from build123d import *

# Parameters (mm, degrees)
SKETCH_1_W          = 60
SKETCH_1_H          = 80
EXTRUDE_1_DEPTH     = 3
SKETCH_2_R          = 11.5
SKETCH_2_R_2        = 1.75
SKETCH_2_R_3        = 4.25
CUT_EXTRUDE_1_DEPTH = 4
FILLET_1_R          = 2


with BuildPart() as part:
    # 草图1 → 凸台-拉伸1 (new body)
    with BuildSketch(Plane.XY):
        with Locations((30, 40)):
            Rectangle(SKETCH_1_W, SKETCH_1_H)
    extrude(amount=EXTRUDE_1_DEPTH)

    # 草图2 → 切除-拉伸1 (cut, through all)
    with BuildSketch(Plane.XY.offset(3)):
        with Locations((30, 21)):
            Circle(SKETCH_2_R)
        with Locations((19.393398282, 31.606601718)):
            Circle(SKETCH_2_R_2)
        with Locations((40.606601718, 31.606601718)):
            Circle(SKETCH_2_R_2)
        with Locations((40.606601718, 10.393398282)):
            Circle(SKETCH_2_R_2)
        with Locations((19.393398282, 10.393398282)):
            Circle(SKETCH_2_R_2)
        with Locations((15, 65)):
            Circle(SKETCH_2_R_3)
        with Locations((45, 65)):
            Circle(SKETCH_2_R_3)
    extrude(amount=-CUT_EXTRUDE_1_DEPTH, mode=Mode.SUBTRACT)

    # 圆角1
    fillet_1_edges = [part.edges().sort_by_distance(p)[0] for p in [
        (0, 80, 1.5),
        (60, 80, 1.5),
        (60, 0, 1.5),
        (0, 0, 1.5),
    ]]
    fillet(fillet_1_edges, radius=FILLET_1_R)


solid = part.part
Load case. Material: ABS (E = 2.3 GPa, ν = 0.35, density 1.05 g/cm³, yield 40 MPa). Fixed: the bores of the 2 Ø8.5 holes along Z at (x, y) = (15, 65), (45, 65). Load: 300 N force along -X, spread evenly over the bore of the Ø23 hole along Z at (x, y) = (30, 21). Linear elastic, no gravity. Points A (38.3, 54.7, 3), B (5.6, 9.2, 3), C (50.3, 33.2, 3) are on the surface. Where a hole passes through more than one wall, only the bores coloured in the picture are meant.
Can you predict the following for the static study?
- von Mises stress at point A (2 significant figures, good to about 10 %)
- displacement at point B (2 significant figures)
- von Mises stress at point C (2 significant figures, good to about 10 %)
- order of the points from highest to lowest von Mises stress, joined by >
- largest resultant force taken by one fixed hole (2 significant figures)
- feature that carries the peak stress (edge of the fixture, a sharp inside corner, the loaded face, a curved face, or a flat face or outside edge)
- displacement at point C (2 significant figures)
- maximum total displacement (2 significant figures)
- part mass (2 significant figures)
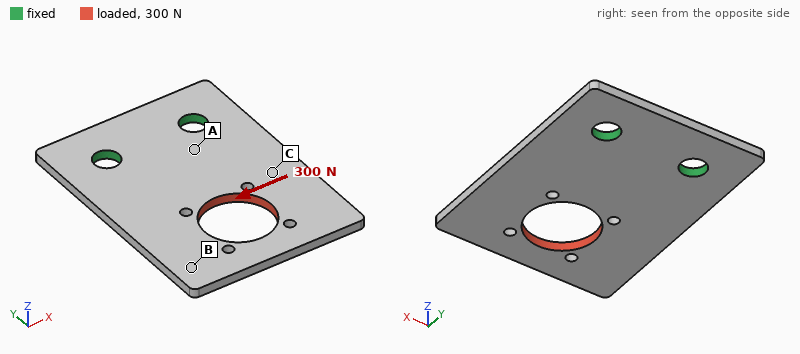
5.7 MPa
0.33 mm
3.1 MPa
A > C > B
380 N
a curved face
0.16 mm
0.39 mm
13 g
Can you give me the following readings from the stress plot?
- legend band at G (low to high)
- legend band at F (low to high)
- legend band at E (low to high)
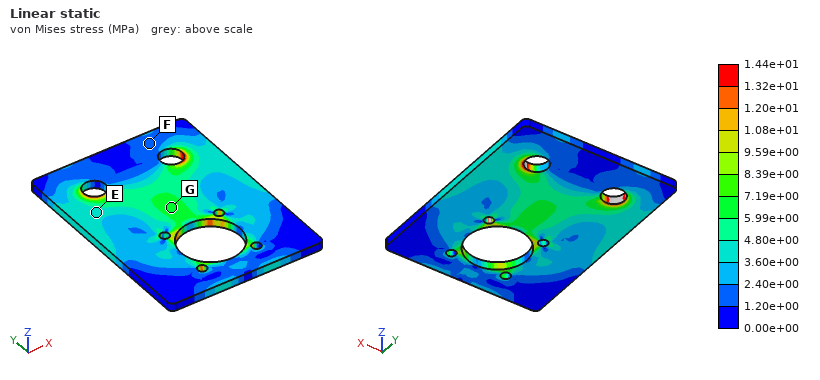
5.99e+00 to 7.19e+00 MPa
1.20e+00 to 2.40e+00 MPa
3.60e+00 to 4.80e+00 MPa
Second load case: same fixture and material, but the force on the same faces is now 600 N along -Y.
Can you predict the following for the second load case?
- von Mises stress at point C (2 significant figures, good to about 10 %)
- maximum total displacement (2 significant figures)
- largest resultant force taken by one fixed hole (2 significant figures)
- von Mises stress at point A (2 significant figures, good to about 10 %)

4.4 MPa
0.17 mm
300 N
3.4 MPa
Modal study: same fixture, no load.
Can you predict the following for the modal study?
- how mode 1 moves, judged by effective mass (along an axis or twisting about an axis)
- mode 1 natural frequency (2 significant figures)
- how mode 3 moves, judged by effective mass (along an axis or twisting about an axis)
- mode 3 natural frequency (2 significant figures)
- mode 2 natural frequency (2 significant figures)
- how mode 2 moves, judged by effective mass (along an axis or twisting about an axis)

along Z
200 Hz
along Z
1000 Hz
420 Hz
twisting about Y
